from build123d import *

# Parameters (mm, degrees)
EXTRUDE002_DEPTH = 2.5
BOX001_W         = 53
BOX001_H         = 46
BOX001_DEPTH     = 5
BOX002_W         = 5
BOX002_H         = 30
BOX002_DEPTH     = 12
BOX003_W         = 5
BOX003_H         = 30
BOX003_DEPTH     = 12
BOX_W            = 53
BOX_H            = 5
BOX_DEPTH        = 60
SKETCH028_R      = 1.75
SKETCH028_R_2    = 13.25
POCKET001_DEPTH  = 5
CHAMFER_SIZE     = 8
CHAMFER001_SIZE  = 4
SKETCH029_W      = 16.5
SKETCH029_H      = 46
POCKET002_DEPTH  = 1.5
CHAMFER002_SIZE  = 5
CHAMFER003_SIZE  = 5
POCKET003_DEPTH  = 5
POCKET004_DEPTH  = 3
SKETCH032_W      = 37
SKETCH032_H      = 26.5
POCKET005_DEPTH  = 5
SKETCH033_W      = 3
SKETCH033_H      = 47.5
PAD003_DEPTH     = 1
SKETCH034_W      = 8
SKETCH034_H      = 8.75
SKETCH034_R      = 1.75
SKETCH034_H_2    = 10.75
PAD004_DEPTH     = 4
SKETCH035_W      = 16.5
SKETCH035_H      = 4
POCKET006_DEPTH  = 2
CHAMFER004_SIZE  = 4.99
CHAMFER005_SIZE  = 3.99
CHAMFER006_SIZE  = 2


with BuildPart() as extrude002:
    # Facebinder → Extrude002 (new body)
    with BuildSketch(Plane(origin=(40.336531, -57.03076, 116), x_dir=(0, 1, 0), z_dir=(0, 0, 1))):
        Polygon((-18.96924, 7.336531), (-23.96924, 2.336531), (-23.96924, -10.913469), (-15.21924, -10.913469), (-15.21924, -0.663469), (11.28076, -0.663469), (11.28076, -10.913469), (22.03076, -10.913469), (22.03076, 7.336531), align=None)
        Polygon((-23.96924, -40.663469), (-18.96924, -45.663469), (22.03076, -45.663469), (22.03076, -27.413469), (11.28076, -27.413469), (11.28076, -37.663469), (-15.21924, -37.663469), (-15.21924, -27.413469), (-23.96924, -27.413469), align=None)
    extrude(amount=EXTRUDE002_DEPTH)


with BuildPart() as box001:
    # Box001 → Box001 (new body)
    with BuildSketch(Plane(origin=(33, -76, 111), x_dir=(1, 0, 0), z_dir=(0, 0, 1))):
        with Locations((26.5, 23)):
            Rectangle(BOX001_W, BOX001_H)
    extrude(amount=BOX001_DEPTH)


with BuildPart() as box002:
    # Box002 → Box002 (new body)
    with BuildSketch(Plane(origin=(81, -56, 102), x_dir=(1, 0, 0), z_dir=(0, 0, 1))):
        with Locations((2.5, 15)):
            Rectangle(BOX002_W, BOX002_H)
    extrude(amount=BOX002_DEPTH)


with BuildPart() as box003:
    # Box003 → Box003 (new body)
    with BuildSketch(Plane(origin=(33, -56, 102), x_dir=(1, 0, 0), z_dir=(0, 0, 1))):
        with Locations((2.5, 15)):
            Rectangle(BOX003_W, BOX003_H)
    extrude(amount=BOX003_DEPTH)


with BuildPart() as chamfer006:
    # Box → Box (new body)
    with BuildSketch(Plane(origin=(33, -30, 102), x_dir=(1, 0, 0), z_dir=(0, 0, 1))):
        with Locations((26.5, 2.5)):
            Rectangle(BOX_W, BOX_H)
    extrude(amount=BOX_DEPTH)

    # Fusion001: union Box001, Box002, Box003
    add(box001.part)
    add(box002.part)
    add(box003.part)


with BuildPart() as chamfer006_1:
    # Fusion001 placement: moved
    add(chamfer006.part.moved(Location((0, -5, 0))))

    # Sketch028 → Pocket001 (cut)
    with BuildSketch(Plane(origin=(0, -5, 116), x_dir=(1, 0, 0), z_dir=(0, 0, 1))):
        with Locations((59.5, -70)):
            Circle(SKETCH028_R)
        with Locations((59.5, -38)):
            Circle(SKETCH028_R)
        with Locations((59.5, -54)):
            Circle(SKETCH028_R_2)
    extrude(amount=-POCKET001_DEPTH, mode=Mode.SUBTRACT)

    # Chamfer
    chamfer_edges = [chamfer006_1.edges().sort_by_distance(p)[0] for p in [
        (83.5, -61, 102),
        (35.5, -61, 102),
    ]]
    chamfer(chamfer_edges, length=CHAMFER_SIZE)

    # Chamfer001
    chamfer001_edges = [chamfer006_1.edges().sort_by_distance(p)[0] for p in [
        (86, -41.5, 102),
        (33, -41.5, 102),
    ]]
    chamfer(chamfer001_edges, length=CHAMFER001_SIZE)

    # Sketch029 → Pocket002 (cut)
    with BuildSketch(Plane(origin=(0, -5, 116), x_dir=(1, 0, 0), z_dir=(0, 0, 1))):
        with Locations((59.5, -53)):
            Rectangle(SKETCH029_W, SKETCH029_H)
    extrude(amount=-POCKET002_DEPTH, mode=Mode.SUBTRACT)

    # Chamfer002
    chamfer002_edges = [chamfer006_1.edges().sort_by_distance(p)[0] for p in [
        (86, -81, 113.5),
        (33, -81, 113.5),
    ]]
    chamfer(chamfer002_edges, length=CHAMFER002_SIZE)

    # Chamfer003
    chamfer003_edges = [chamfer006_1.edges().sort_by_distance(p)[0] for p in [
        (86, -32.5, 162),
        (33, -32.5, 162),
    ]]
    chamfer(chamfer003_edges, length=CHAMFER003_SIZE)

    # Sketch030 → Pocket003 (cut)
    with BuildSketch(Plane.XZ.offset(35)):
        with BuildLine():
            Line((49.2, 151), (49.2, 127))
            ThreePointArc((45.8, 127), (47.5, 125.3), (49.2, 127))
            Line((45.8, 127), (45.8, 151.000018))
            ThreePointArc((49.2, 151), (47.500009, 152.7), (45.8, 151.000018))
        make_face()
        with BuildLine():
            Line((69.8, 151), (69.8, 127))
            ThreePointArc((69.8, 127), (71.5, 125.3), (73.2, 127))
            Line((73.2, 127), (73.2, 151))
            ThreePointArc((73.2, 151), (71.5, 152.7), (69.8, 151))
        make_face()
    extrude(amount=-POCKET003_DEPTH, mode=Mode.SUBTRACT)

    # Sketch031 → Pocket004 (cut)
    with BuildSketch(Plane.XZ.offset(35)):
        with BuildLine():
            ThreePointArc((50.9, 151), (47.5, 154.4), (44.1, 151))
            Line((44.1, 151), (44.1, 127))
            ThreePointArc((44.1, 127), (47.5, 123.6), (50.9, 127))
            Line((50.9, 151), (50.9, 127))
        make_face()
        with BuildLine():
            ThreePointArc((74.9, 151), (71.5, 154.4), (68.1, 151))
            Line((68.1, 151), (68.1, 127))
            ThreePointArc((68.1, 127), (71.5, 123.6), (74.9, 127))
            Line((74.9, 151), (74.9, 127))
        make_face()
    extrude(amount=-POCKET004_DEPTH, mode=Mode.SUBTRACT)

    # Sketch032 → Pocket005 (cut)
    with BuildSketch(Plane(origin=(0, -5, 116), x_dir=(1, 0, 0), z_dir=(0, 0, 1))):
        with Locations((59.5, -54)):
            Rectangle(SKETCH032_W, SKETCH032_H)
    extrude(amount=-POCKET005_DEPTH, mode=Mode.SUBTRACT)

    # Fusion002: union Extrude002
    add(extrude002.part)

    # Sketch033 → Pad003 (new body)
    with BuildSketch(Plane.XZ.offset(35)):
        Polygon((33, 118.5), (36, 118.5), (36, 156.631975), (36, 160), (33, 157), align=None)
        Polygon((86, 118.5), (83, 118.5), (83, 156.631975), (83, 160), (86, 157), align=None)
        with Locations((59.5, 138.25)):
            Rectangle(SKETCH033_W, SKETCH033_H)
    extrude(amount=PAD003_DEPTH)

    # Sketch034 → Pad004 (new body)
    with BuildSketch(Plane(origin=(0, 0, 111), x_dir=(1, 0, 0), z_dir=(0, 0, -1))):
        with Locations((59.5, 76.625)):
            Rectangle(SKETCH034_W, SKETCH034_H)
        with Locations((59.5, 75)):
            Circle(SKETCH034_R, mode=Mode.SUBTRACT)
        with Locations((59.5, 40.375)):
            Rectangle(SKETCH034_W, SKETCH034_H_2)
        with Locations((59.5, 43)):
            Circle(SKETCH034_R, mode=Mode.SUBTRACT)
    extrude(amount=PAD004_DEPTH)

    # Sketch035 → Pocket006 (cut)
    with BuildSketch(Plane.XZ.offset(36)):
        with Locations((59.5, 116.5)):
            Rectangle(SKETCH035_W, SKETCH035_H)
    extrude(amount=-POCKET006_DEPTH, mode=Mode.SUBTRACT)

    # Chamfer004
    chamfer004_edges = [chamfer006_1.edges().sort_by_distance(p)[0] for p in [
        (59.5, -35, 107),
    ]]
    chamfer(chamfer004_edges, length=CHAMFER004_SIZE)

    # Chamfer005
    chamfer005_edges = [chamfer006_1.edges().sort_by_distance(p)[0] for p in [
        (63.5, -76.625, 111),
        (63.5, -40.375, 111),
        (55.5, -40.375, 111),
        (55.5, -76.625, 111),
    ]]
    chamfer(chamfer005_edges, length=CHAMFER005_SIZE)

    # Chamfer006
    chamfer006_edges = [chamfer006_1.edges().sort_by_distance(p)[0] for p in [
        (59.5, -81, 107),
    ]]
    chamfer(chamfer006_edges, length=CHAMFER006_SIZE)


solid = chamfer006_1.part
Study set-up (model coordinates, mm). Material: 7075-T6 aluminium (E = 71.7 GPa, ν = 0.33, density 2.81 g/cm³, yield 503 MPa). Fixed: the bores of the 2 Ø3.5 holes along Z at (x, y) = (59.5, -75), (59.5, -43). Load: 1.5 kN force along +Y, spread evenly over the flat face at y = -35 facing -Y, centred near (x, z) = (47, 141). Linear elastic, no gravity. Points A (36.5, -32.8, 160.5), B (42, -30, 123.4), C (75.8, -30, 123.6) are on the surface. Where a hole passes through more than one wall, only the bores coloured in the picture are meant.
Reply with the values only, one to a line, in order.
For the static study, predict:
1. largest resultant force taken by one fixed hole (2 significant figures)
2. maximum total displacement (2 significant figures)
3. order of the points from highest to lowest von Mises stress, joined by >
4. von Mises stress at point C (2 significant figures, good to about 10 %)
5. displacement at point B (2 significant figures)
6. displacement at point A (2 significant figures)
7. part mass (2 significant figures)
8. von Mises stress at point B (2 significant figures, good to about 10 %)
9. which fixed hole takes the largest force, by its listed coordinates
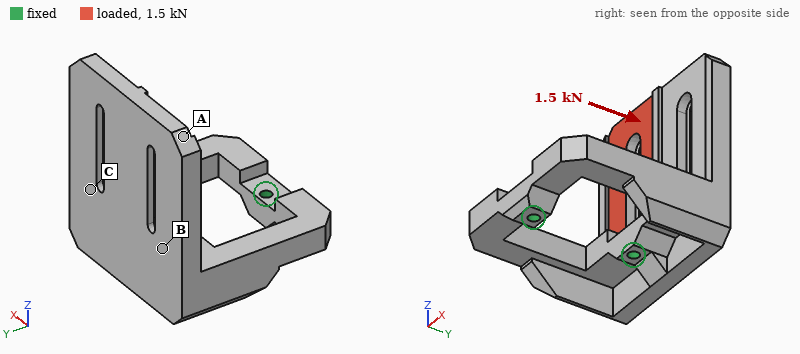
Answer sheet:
1.3 kN
0.95 mm
B > C > A
87 MPa
0.15 mm
0.92 mm
74 g
140 MPa
(59.5, -43)
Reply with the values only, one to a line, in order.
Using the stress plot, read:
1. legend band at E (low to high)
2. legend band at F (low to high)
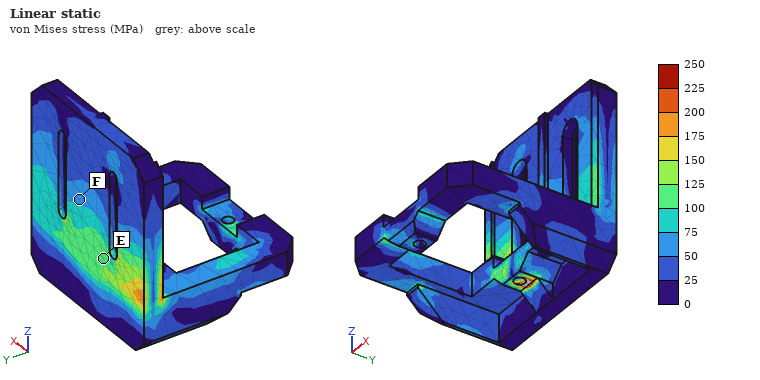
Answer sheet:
100 to 125 MPa
50 to 75 MPa
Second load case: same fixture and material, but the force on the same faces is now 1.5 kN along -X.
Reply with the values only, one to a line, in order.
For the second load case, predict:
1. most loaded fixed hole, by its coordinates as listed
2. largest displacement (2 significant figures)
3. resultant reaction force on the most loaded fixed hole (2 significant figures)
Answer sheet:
(59.5, -43)
0.45 mm
1.7 kN
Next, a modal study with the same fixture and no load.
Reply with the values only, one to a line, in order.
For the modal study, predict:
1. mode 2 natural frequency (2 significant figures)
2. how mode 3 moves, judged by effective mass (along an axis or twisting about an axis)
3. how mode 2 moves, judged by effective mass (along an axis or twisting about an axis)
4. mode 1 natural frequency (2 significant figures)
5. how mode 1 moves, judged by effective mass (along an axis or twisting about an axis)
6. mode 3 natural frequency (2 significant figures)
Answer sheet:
1800 Hz
twisting about Z
along X
1600 Hz
along Y
3400 Hz
